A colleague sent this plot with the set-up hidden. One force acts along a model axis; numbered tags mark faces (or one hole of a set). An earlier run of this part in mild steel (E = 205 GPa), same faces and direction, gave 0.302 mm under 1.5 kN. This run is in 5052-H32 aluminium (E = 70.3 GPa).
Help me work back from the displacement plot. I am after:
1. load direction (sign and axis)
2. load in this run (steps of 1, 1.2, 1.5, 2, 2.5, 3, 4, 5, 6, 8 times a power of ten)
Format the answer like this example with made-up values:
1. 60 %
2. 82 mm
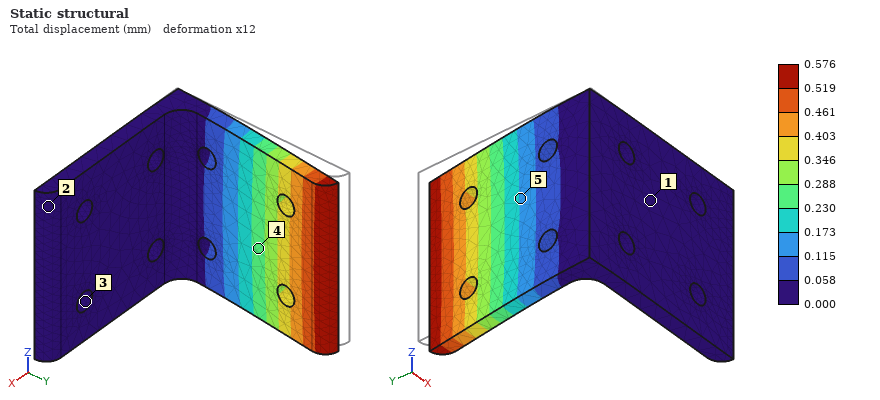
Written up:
1. +X
2. 1 kN
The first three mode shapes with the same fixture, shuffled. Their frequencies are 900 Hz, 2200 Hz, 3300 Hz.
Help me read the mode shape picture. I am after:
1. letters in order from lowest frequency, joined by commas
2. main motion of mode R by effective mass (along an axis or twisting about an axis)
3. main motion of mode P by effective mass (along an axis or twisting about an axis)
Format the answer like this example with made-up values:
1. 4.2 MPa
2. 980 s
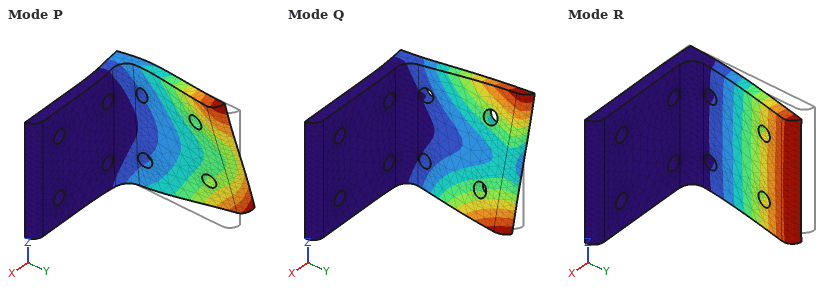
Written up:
1. R, Q, P
2. along X
3. along Z
